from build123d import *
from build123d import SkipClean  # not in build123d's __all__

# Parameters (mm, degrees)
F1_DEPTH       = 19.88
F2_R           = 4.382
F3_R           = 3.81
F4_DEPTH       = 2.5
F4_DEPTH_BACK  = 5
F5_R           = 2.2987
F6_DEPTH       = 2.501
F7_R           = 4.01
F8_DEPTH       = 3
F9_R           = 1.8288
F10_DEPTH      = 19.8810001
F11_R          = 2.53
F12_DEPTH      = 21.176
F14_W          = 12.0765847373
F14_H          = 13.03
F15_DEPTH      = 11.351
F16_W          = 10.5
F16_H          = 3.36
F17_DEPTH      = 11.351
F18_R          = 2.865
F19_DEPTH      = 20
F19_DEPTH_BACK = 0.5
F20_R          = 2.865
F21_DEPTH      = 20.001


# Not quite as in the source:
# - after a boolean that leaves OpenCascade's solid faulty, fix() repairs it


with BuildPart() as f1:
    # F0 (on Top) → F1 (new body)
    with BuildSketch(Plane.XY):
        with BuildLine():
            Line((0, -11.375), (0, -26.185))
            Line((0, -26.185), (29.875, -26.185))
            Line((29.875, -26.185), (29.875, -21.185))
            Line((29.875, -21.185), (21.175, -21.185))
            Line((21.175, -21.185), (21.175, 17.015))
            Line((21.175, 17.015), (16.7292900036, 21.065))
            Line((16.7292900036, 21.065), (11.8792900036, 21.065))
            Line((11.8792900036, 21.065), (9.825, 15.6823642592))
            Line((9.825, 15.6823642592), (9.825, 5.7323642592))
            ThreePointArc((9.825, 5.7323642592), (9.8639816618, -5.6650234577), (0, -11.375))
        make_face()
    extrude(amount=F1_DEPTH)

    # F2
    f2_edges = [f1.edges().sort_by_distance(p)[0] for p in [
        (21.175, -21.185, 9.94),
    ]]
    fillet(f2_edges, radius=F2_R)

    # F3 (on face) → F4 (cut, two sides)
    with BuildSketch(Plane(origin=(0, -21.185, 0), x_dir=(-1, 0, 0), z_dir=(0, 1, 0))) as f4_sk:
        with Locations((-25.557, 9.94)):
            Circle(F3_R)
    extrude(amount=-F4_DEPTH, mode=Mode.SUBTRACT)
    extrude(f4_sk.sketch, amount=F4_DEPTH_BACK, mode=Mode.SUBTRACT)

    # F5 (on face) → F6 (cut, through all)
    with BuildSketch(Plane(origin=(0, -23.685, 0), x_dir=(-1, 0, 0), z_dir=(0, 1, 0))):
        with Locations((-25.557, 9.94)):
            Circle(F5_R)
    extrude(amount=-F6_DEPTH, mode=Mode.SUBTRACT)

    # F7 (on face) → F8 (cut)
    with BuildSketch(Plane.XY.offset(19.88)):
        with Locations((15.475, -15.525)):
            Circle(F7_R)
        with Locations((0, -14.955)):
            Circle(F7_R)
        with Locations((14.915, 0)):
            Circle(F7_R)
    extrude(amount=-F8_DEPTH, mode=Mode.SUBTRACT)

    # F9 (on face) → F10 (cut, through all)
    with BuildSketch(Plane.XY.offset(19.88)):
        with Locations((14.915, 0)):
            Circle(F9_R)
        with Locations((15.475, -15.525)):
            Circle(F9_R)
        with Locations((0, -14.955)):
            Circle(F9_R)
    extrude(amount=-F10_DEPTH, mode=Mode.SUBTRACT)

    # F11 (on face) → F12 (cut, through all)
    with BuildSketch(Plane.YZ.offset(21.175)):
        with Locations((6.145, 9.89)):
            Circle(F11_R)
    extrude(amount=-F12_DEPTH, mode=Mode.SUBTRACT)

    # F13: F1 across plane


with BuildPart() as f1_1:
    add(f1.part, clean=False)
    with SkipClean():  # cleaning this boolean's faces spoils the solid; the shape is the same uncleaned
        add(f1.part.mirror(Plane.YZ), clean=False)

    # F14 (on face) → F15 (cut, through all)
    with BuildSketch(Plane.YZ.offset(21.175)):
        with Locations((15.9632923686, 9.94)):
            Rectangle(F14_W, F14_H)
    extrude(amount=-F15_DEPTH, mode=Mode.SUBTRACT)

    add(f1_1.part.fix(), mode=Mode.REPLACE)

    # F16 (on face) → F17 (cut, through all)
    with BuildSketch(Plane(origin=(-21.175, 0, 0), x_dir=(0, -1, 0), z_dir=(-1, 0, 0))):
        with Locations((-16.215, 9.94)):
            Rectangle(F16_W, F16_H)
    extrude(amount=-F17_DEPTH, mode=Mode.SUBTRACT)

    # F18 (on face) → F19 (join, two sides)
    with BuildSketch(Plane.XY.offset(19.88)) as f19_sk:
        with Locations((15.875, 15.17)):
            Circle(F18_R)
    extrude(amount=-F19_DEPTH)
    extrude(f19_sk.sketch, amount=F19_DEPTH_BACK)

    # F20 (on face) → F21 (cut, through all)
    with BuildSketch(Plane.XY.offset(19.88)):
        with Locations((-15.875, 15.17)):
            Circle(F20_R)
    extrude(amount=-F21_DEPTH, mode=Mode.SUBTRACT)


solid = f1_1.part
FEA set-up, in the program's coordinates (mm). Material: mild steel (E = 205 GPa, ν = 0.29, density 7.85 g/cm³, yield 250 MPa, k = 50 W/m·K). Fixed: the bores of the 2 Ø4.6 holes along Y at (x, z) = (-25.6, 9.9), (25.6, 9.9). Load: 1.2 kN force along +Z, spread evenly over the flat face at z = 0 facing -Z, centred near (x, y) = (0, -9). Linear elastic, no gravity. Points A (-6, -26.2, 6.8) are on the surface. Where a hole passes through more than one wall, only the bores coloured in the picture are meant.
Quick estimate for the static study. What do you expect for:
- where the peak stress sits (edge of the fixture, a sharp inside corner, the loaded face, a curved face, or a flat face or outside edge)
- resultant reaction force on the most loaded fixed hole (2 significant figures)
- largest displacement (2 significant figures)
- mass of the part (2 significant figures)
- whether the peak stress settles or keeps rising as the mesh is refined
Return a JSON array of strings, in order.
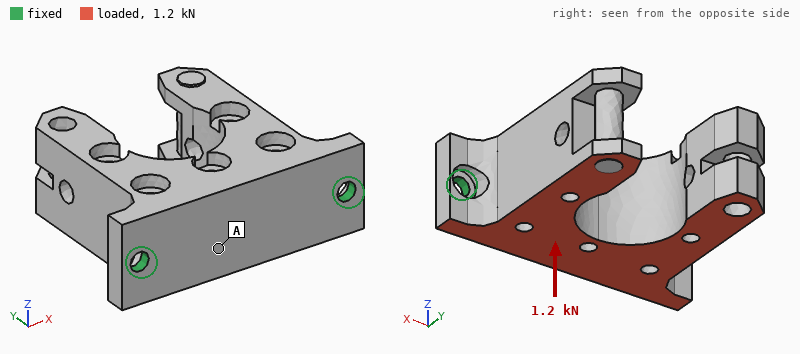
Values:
["edge of the fixture", "600 N", "92 µm", "190 g", "keeps rising"]
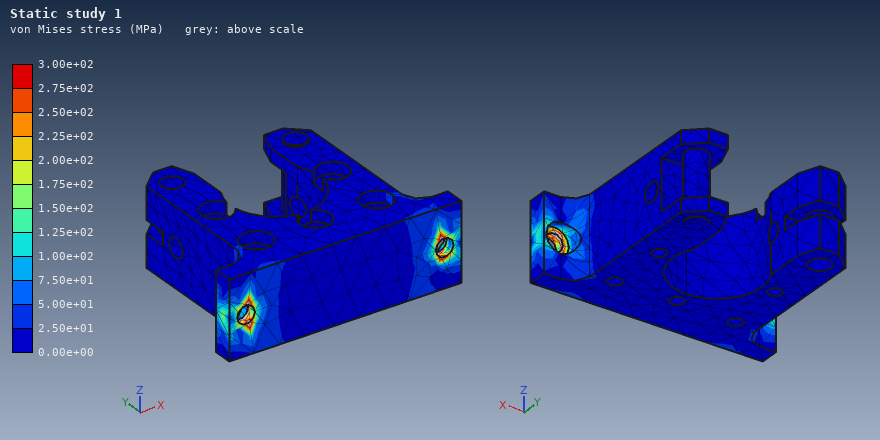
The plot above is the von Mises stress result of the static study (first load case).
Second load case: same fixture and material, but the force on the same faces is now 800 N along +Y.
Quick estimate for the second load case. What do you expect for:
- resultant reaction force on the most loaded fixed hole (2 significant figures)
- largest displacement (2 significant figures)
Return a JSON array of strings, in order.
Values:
["480 N", "37 µm"]
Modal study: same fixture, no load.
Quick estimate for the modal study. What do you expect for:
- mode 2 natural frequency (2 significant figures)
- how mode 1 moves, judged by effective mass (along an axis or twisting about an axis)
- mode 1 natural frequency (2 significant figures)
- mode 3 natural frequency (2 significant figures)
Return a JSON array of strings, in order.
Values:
["6400 Hz", "along Z", "1800 Hz", "6600 Hz"]
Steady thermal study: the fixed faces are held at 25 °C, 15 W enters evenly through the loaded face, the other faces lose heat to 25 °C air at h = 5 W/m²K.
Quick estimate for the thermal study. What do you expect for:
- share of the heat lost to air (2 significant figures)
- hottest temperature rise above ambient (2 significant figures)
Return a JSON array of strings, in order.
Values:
["5.6 %", "28 K"]
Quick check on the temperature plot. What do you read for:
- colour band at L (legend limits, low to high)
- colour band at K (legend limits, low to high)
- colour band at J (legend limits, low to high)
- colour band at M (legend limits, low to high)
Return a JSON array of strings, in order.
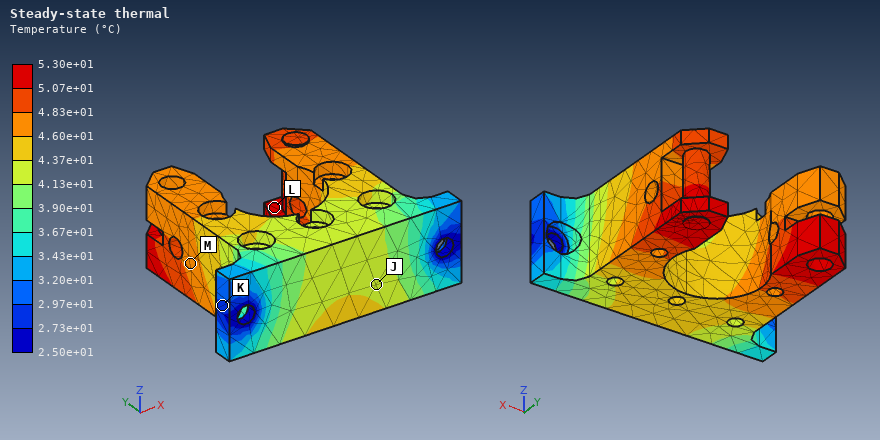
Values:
["5.07e+01 to 5.30e+01 °C", "2.73e+01 to 2.97e+01 °C", "4.13e+01 to 4.37e+01 °C", "4.60e+01 to 4.83e+01 °C"]
